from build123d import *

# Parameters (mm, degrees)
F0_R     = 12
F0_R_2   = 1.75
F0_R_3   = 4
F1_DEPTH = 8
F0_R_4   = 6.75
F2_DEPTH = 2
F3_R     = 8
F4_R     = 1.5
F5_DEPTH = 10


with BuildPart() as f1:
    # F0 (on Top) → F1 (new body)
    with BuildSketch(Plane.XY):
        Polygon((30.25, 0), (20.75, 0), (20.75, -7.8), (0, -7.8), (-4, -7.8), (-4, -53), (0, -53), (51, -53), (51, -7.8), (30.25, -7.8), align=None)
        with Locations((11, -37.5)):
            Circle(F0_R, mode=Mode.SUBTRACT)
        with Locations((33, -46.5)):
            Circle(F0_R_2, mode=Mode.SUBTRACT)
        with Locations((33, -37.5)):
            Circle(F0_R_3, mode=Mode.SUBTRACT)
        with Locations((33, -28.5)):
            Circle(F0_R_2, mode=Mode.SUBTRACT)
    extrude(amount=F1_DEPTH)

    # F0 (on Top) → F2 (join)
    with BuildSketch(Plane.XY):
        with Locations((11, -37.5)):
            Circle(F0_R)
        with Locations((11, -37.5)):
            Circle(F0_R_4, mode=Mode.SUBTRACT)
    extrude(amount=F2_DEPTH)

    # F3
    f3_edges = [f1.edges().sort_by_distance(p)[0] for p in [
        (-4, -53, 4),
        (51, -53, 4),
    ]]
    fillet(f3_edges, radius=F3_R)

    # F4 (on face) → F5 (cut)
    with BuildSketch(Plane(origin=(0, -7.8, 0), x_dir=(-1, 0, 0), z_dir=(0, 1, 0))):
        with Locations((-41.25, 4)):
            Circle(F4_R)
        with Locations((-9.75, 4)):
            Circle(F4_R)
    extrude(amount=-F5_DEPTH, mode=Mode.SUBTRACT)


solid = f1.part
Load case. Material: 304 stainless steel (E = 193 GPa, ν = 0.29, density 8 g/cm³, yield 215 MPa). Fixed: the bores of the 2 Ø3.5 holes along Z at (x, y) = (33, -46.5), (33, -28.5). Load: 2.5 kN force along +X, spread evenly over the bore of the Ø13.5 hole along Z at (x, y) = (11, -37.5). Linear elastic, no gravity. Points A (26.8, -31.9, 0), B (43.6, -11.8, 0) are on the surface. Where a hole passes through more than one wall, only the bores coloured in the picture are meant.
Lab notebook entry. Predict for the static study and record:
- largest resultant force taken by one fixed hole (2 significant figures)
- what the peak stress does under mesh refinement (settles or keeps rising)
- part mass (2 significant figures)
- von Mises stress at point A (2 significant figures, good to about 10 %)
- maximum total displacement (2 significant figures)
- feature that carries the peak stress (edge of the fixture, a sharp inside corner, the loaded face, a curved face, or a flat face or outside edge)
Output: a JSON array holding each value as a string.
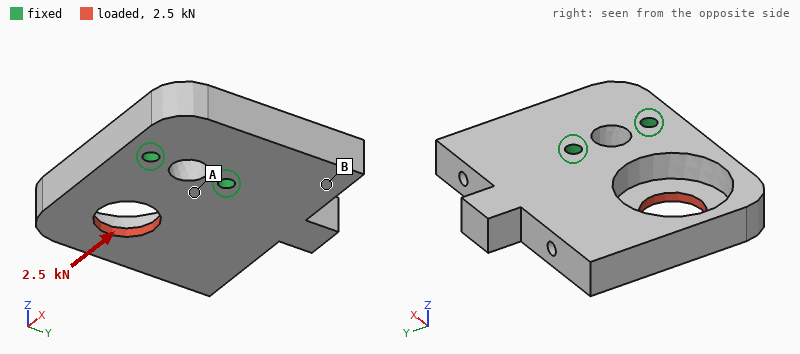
["1.3 kN", "keeps rising", "130 g", "31 MPa", "17 µm", "edge of the fixture"]
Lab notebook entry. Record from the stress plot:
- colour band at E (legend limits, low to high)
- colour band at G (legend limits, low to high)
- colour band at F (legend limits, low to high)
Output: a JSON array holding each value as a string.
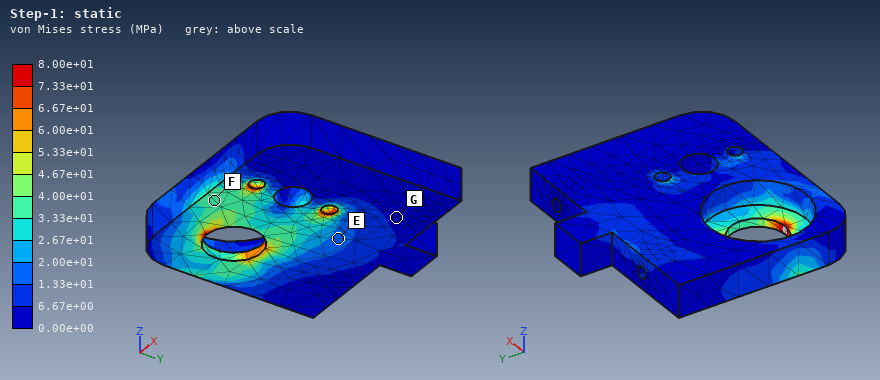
["1.33e+01 to 2.00e+01 MPa", "0.00e+00 to 6.67e+00 MPa", "3.33e+01 to 4.00e+01 MPa"]
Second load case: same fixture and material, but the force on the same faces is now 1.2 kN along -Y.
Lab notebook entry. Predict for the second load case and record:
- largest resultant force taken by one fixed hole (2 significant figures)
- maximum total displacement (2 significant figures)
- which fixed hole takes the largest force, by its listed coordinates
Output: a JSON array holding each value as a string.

["1.4 kN", "9.2 µm", "(33, -28.5)"]
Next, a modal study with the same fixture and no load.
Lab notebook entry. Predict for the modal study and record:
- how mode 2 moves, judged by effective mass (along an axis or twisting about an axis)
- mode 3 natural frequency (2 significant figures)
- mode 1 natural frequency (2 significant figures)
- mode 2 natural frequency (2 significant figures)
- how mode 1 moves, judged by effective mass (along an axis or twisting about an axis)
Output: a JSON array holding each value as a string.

["twisting about X", "8000 Hz", "3800 Hz", "6500 Hz", "along Z"]
